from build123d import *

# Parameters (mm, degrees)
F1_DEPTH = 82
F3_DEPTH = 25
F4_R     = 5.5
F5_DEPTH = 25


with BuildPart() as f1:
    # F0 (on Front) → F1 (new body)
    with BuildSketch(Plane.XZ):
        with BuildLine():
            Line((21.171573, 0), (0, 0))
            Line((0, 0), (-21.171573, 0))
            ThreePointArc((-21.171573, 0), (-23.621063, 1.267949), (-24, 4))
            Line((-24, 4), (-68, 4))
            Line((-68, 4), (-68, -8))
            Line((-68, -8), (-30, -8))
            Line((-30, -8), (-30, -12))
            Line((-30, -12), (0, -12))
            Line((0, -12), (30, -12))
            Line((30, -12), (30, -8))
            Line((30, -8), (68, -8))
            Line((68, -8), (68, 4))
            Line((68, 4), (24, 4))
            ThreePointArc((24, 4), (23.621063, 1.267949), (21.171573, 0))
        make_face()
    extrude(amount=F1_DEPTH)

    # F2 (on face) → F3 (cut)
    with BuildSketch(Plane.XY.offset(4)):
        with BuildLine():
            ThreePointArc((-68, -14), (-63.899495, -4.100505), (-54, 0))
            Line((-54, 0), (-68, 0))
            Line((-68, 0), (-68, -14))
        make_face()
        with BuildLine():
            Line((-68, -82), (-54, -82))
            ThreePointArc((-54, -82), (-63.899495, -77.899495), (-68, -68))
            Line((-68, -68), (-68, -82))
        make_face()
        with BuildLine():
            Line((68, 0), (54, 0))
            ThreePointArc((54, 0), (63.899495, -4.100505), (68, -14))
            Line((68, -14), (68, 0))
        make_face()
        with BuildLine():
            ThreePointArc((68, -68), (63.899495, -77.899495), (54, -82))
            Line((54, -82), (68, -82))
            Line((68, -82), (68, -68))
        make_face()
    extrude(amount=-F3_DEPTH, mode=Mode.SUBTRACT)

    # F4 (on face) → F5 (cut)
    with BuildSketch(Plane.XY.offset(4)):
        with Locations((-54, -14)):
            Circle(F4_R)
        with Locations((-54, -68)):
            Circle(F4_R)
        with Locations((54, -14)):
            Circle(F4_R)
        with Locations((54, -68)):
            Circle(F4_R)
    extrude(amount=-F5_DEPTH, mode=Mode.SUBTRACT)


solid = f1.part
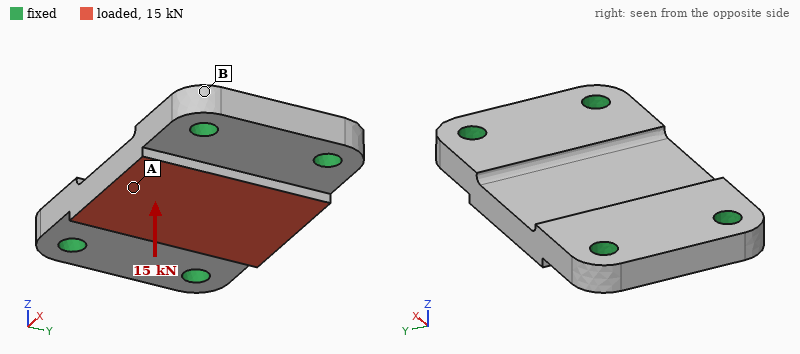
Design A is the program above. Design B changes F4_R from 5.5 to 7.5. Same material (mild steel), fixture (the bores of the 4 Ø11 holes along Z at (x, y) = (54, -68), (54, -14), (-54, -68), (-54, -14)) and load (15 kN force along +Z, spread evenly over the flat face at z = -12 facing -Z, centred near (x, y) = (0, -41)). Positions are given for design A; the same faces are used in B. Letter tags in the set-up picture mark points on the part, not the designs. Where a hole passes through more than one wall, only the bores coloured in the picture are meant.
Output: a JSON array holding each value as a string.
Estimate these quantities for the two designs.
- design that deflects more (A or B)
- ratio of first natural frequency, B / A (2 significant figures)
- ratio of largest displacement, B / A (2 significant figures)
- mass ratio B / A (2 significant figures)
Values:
["A", "1.1", "0.84", "0.97"]
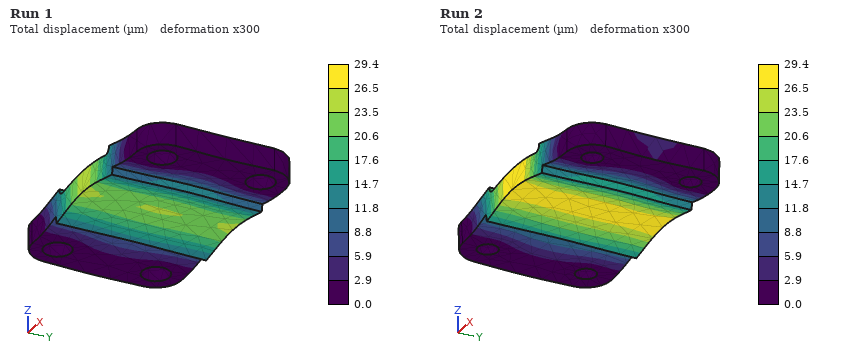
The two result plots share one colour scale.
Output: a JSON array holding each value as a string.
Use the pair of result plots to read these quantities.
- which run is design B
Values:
["Run 1"]
